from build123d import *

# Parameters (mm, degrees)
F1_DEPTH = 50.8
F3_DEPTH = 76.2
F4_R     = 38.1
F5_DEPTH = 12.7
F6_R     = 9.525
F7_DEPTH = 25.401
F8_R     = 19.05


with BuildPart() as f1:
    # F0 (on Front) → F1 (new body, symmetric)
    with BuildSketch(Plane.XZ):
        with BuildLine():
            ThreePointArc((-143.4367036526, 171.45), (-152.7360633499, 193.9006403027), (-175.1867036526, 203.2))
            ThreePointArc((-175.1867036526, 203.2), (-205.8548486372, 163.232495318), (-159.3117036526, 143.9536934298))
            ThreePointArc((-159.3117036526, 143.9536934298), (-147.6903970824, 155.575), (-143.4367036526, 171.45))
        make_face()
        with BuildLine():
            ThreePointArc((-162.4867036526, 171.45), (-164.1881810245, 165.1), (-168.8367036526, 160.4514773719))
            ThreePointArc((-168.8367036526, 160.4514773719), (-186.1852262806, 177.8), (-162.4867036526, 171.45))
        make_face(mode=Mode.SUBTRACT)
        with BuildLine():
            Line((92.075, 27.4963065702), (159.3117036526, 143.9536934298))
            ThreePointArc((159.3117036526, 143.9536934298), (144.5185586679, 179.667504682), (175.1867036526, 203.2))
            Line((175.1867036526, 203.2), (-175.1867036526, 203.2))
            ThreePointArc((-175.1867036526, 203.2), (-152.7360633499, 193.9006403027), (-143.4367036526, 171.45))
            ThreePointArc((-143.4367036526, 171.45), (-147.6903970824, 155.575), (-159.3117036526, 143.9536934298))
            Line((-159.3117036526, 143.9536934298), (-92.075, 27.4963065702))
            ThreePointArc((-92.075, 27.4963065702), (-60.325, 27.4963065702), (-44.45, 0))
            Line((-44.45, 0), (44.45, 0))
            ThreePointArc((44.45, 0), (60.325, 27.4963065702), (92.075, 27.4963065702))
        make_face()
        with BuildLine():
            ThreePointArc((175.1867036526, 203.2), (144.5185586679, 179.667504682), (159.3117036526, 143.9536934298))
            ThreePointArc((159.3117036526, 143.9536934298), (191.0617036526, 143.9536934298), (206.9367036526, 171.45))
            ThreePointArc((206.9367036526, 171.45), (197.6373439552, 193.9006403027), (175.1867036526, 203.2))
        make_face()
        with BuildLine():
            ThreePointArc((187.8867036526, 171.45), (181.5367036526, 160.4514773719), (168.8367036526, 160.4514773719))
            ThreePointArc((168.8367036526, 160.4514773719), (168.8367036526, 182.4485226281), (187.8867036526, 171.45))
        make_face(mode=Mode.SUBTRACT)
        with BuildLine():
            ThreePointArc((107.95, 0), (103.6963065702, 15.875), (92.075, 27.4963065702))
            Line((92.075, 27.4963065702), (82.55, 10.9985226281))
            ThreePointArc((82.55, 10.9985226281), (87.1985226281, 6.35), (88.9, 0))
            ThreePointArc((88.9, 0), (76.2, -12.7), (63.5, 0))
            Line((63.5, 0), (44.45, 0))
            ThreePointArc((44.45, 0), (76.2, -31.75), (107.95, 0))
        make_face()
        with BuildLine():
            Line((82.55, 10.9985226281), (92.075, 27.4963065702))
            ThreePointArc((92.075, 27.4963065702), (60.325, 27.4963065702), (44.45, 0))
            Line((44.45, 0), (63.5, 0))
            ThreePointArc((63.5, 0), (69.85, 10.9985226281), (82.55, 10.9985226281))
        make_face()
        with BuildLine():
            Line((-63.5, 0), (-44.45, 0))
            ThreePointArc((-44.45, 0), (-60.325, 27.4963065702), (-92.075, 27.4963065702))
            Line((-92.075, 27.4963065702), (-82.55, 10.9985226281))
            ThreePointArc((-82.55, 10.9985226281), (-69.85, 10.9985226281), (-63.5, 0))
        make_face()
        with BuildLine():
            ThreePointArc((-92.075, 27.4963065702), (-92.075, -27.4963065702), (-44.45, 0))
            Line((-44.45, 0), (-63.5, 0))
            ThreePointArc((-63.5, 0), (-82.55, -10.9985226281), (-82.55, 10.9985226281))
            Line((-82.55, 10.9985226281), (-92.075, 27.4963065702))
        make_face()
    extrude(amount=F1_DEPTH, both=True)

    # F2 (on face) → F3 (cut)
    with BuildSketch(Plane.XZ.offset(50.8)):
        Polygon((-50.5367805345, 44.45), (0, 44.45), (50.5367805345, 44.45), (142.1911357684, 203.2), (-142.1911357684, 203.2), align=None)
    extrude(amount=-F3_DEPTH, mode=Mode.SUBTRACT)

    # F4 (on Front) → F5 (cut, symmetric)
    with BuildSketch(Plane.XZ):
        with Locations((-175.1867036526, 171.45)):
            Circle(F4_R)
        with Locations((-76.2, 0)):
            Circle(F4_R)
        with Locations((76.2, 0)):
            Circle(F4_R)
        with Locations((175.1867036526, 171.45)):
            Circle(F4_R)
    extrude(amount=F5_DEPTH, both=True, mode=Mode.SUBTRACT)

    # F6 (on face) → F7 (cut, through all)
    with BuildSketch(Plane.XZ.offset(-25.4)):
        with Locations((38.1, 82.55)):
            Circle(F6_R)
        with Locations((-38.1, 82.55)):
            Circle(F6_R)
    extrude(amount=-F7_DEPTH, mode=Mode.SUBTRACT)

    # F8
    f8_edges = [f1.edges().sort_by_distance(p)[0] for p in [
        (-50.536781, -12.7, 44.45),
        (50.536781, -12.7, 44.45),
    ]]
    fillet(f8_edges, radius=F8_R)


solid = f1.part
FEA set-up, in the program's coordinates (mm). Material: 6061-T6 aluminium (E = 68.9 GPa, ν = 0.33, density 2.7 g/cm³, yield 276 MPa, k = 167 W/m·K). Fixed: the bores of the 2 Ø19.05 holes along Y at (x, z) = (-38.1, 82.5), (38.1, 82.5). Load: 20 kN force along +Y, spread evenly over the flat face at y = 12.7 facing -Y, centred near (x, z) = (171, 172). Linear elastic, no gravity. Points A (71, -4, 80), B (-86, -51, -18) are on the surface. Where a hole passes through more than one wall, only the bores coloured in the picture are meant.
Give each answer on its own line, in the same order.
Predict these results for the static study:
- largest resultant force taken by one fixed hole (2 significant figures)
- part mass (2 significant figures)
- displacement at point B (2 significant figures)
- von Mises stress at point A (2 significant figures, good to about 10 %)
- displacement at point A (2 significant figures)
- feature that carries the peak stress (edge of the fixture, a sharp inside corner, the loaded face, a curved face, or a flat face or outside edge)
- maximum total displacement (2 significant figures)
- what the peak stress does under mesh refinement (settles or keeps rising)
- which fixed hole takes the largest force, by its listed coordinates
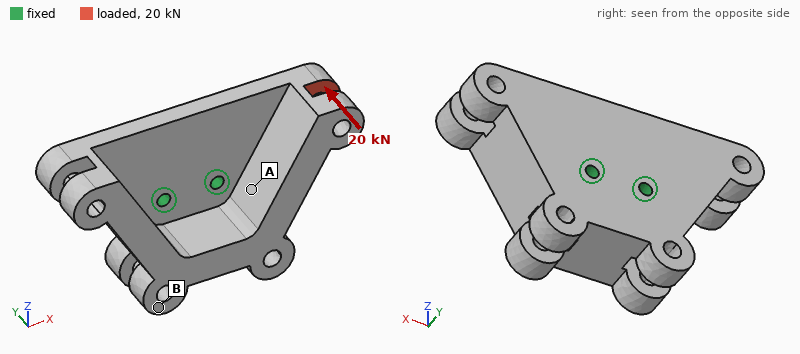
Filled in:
41 kN
9.3 kg
0.32 mm
31 MPa
0.15 mm
edge of the fixture
0.79 mm
keeps rising
(38.1, 82.5)
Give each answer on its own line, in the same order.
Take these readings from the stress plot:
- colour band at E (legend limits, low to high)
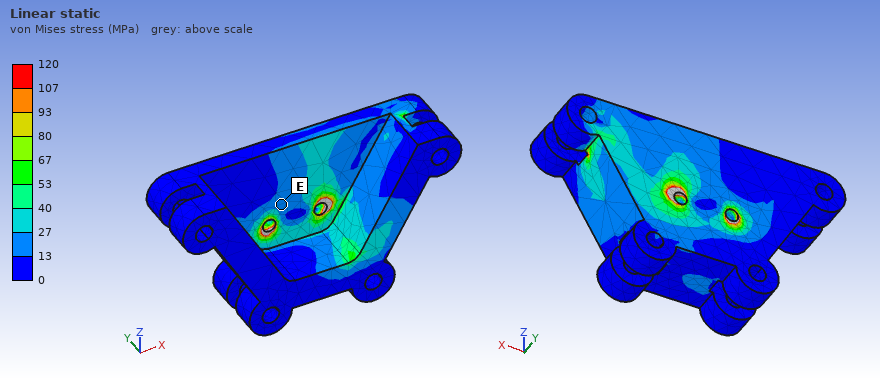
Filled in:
13 to 27 MPa
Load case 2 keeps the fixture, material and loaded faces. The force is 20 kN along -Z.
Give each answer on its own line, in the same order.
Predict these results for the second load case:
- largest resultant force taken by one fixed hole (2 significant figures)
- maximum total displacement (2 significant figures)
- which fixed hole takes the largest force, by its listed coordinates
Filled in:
48 kN
0.22 mm
(38.1, 82.5)
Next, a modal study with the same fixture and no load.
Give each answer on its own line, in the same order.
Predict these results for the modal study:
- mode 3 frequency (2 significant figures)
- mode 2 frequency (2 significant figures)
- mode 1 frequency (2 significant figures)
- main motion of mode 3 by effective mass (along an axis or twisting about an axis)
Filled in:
1100 Hz
820 Hz
630 Hz
twisting about Y
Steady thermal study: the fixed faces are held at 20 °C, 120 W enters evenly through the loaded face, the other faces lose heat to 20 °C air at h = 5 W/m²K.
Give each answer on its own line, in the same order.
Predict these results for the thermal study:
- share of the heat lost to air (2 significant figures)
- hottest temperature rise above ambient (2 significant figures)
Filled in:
7.9 %
35 K
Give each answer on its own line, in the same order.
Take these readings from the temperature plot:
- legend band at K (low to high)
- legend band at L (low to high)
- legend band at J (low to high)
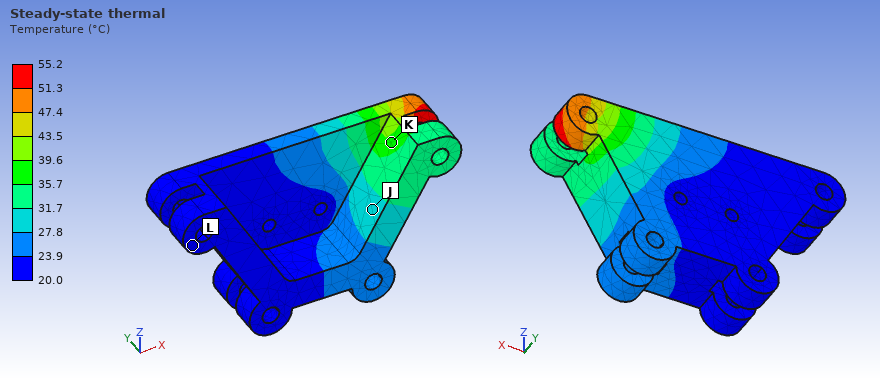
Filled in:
35.7 to 39.6 °C
20.0 to 23.9 °C
27.8 to 31.7 °C
